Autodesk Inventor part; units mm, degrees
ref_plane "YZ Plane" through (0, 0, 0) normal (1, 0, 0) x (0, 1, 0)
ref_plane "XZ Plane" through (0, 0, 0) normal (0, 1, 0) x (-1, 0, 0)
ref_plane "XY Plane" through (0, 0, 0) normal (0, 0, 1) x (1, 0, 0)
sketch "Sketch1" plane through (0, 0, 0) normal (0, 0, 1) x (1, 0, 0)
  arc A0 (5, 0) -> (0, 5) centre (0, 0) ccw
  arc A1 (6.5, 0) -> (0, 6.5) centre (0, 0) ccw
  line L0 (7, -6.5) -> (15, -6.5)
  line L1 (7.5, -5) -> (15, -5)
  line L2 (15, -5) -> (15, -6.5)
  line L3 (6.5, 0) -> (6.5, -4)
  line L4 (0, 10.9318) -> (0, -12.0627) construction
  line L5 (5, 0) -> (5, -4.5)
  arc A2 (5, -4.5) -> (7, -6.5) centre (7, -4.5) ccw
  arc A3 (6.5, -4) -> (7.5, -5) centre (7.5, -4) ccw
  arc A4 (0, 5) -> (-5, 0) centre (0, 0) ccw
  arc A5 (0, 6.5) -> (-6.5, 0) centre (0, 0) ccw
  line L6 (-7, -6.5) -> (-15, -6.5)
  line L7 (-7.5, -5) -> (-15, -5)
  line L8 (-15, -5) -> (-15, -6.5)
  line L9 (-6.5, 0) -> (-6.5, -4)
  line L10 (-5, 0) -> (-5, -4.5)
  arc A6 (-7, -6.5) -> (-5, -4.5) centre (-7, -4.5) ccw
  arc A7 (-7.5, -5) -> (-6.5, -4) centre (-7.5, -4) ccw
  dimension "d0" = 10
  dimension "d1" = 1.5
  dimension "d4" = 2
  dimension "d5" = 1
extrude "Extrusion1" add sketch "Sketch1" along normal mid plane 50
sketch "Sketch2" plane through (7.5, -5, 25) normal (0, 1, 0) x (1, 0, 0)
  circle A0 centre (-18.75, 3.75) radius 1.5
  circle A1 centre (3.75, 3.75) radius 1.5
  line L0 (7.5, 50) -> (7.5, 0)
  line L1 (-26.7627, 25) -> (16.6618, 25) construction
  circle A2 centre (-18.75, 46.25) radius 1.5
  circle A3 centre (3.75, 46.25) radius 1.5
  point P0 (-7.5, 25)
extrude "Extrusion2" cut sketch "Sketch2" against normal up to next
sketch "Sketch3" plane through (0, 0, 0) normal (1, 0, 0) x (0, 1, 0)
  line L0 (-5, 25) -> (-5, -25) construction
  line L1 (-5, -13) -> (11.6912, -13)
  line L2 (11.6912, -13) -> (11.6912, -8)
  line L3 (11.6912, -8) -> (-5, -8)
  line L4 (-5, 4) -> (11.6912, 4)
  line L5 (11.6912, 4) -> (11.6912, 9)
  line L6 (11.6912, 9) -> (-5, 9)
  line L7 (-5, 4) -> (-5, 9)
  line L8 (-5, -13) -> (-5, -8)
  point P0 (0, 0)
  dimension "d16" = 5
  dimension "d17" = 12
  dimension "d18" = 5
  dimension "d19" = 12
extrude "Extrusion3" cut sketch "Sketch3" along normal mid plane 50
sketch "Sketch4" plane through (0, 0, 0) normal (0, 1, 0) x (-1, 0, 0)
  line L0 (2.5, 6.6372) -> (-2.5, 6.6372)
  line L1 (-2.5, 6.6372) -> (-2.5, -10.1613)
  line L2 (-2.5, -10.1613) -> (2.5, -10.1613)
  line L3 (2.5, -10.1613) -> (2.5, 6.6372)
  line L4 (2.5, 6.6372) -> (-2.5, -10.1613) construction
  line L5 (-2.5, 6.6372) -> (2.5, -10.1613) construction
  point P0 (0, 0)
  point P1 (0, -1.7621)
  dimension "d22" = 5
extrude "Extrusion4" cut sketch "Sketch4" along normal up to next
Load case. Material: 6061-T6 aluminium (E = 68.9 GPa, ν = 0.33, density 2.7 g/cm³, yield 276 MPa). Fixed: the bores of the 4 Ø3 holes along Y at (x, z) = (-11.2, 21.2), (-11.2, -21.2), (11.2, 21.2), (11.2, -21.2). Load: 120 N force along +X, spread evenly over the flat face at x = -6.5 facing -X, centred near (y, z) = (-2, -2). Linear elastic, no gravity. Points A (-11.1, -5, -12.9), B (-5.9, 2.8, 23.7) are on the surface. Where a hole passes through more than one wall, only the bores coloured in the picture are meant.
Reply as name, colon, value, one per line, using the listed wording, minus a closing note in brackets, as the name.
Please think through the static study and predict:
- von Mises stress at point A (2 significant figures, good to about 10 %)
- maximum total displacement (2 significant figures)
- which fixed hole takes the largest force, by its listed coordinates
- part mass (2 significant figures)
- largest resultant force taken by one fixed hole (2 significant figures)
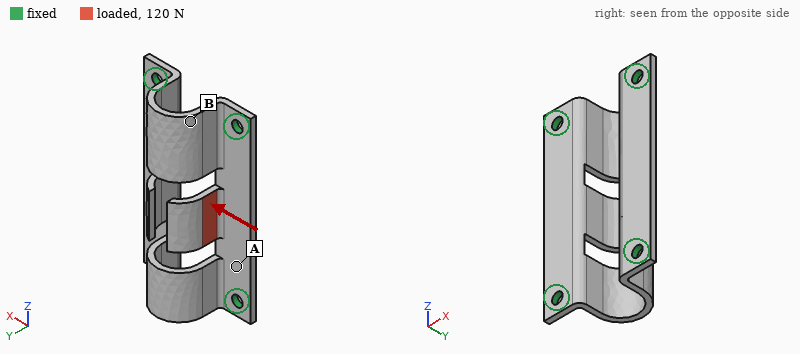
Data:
von Mises stress at point A: 55 MPa
maximum total displacement: 0.20 mm
which fixed hole takes the largest force, by its listed coordinates: (-11.2, -21.2)
part mass: 8.0 g
largest resultant force taken by one fixed hole: 64 N
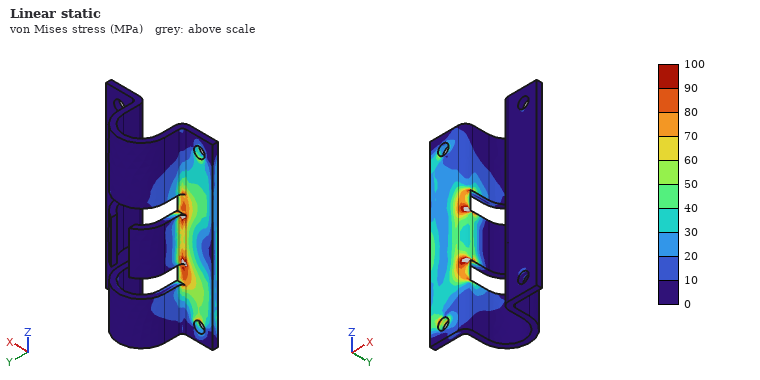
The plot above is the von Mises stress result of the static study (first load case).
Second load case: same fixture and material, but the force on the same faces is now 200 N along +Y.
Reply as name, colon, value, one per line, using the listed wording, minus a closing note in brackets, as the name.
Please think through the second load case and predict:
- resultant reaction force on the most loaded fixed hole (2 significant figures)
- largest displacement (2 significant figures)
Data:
resultant reaction force on the most loaded fixed hole: 99 N
largest displacement: 0.20 mm
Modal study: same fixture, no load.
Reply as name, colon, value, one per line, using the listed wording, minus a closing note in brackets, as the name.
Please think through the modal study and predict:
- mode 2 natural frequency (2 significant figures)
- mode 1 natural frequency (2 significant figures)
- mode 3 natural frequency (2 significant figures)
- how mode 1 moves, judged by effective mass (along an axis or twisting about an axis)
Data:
mode 2 natural frequency: 4400 Hz
mode 1 natural frequency: 3800 Hz
mode 3 natural frequency: 4700 Hz
how mode 1 moves, judged by effective mass: along Y
